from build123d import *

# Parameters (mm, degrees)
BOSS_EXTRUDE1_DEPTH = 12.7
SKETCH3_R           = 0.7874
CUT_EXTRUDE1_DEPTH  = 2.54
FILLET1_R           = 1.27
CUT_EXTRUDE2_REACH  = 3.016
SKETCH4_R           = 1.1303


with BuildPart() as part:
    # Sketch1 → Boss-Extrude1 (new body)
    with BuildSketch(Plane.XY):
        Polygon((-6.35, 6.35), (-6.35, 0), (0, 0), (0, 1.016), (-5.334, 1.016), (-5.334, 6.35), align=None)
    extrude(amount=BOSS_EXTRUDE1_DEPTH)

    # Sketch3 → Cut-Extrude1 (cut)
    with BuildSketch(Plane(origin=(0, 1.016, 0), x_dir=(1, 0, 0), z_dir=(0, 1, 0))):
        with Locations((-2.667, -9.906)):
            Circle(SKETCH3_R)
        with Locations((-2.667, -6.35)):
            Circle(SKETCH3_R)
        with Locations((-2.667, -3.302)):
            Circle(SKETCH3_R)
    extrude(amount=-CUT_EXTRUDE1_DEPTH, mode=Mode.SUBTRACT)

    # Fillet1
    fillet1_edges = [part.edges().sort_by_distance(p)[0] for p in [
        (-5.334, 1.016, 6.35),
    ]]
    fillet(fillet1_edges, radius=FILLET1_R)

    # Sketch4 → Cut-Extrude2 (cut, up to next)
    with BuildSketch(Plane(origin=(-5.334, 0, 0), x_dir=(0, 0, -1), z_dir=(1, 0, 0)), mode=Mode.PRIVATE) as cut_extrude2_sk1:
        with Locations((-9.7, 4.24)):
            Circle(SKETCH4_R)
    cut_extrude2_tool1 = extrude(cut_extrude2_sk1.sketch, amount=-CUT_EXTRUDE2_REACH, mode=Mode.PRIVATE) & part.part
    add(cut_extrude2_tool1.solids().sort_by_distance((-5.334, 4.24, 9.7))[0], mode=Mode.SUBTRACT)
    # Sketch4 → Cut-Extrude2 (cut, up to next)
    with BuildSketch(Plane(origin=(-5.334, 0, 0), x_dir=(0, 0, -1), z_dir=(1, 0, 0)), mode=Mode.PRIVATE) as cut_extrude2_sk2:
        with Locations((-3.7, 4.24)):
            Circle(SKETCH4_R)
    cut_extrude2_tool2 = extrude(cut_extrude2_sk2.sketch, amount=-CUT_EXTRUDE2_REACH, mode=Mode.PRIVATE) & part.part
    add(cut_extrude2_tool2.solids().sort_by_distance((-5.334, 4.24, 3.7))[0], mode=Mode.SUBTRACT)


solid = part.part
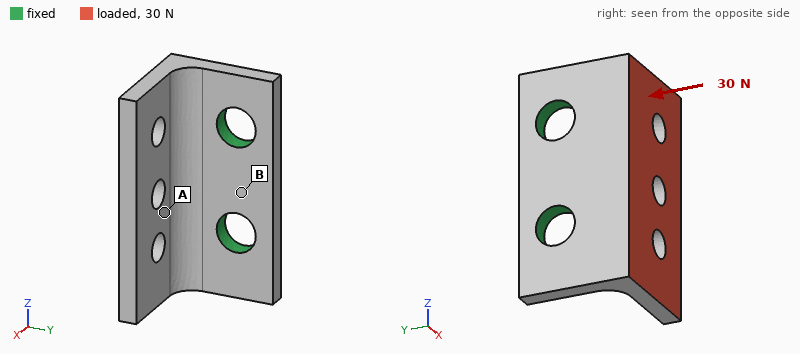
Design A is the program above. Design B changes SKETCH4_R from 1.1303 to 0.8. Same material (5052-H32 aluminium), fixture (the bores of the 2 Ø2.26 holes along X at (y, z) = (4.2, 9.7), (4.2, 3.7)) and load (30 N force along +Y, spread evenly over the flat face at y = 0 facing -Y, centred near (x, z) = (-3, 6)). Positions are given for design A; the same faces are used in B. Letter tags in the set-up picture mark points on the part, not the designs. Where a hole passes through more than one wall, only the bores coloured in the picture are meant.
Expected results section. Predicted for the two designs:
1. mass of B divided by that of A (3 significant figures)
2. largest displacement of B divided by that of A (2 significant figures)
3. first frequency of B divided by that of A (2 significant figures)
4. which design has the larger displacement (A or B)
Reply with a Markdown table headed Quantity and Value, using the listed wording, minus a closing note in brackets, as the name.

| Quantity | Value |
|---|---|
| mass of B divided by that of A | 1.03 |
| largest displacement of B divided by that of A | 1.2 |
| first frequency of B divided by that of A | 0.90 |
| which design has the larger displacement | B |
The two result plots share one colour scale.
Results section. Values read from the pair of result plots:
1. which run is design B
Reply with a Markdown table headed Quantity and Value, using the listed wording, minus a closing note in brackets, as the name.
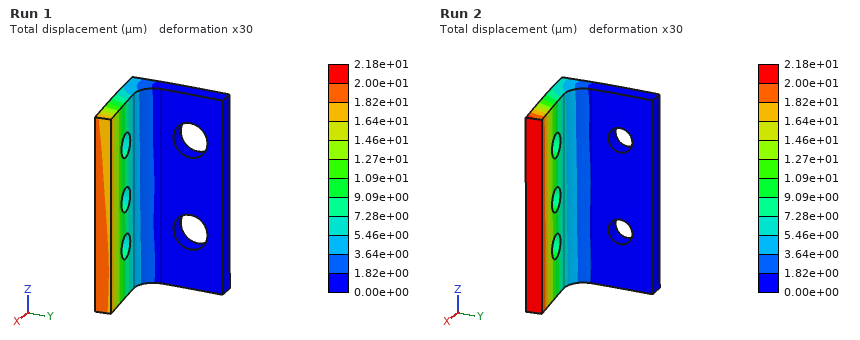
| Quantity | Value |
|---|---|
| which run is design B | Run 2 |
